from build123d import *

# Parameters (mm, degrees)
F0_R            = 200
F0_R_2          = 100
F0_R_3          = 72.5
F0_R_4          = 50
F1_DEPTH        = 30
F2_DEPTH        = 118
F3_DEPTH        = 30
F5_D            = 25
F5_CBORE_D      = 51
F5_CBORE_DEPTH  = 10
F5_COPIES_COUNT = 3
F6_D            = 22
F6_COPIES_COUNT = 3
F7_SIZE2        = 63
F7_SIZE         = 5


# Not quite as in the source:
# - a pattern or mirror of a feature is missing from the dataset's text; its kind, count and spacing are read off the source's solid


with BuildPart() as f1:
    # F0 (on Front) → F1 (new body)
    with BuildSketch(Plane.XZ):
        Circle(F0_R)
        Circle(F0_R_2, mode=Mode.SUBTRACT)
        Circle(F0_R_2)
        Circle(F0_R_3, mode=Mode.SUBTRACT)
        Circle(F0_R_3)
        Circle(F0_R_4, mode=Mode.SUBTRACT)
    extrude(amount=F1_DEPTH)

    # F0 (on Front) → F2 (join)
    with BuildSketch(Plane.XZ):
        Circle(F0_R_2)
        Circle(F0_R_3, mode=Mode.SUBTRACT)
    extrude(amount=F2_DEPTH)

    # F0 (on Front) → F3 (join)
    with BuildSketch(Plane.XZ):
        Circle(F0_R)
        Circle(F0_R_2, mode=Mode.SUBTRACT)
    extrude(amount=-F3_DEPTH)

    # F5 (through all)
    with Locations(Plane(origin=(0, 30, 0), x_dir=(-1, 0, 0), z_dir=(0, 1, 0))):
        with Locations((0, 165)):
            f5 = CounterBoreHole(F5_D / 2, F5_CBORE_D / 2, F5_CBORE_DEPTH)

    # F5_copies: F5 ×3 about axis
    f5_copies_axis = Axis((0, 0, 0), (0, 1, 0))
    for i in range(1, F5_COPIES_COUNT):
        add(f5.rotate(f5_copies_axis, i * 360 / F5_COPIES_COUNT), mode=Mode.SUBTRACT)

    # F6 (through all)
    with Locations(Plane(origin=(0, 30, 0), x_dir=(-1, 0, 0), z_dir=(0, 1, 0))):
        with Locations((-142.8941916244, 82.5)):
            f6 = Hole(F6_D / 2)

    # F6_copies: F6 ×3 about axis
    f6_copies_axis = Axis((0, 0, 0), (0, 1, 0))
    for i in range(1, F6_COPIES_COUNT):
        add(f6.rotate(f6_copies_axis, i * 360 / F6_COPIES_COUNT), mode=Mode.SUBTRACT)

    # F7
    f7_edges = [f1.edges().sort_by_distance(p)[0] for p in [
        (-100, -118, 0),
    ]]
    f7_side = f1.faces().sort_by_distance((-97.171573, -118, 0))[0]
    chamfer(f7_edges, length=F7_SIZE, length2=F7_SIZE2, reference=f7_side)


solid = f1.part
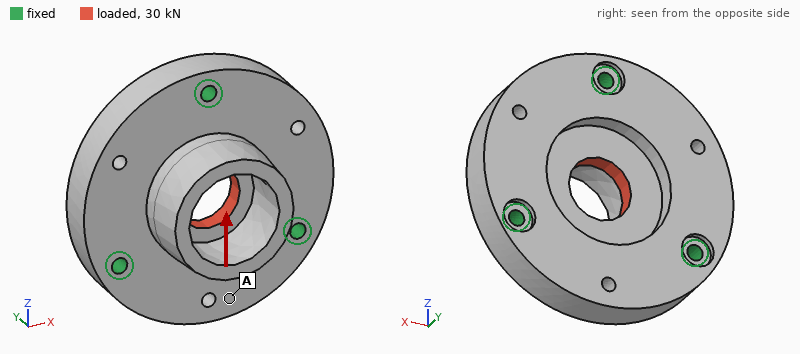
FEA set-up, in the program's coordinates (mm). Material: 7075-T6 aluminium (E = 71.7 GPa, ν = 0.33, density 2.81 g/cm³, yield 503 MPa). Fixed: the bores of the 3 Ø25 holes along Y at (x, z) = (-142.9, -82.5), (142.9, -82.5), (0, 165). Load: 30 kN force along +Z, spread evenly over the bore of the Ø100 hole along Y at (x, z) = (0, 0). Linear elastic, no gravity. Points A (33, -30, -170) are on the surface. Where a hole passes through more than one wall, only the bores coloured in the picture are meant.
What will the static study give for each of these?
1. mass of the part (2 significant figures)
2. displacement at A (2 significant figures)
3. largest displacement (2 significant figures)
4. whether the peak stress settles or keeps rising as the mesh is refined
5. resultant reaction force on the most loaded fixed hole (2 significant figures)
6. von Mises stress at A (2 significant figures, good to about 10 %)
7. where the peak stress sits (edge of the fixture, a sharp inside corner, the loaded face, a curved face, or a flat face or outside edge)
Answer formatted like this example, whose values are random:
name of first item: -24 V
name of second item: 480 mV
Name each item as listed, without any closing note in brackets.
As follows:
mass of the part: 21 kg
displacement at A: 5.1 µm
largest displacement: 7.6 µm
whether the peak stress settles or keeps rising as the mesh is refined: keeps rising
resultant reaction force on the most loaded fixed hole: 10 kN
von Mises stress at A: 1.0 MPa
where the peak stress sits: edge of the fixture
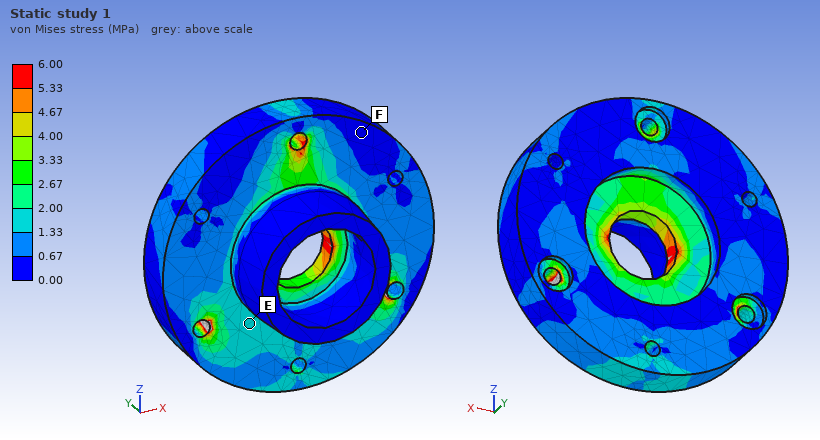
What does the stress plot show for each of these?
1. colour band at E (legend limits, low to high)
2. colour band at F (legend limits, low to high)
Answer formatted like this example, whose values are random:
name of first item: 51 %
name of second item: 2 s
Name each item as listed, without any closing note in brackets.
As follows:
colour band at E: 1.33 to 2.00 MPa
colour band at F: 0.00 to 0.67 MPa
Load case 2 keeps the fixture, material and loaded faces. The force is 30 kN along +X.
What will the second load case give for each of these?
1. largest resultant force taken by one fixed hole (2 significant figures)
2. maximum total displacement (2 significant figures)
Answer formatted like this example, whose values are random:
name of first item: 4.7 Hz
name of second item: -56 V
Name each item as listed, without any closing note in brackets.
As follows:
largest resultant force taken by one fixed hole: 10 kN
maximum total displacement: 7.3 µm
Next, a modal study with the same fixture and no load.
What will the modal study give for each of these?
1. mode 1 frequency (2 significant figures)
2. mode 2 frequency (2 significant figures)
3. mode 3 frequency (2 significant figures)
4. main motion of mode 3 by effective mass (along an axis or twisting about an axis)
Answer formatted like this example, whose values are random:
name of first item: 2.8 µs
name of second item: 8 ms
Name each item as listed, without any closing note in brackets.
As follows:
mode 1 frequency: 1800 Hz
mode 2 frequency: 1800 Hz
mode 3 frequency: 2100 Hz
main motion of mode 3 by effective mass: along Y
